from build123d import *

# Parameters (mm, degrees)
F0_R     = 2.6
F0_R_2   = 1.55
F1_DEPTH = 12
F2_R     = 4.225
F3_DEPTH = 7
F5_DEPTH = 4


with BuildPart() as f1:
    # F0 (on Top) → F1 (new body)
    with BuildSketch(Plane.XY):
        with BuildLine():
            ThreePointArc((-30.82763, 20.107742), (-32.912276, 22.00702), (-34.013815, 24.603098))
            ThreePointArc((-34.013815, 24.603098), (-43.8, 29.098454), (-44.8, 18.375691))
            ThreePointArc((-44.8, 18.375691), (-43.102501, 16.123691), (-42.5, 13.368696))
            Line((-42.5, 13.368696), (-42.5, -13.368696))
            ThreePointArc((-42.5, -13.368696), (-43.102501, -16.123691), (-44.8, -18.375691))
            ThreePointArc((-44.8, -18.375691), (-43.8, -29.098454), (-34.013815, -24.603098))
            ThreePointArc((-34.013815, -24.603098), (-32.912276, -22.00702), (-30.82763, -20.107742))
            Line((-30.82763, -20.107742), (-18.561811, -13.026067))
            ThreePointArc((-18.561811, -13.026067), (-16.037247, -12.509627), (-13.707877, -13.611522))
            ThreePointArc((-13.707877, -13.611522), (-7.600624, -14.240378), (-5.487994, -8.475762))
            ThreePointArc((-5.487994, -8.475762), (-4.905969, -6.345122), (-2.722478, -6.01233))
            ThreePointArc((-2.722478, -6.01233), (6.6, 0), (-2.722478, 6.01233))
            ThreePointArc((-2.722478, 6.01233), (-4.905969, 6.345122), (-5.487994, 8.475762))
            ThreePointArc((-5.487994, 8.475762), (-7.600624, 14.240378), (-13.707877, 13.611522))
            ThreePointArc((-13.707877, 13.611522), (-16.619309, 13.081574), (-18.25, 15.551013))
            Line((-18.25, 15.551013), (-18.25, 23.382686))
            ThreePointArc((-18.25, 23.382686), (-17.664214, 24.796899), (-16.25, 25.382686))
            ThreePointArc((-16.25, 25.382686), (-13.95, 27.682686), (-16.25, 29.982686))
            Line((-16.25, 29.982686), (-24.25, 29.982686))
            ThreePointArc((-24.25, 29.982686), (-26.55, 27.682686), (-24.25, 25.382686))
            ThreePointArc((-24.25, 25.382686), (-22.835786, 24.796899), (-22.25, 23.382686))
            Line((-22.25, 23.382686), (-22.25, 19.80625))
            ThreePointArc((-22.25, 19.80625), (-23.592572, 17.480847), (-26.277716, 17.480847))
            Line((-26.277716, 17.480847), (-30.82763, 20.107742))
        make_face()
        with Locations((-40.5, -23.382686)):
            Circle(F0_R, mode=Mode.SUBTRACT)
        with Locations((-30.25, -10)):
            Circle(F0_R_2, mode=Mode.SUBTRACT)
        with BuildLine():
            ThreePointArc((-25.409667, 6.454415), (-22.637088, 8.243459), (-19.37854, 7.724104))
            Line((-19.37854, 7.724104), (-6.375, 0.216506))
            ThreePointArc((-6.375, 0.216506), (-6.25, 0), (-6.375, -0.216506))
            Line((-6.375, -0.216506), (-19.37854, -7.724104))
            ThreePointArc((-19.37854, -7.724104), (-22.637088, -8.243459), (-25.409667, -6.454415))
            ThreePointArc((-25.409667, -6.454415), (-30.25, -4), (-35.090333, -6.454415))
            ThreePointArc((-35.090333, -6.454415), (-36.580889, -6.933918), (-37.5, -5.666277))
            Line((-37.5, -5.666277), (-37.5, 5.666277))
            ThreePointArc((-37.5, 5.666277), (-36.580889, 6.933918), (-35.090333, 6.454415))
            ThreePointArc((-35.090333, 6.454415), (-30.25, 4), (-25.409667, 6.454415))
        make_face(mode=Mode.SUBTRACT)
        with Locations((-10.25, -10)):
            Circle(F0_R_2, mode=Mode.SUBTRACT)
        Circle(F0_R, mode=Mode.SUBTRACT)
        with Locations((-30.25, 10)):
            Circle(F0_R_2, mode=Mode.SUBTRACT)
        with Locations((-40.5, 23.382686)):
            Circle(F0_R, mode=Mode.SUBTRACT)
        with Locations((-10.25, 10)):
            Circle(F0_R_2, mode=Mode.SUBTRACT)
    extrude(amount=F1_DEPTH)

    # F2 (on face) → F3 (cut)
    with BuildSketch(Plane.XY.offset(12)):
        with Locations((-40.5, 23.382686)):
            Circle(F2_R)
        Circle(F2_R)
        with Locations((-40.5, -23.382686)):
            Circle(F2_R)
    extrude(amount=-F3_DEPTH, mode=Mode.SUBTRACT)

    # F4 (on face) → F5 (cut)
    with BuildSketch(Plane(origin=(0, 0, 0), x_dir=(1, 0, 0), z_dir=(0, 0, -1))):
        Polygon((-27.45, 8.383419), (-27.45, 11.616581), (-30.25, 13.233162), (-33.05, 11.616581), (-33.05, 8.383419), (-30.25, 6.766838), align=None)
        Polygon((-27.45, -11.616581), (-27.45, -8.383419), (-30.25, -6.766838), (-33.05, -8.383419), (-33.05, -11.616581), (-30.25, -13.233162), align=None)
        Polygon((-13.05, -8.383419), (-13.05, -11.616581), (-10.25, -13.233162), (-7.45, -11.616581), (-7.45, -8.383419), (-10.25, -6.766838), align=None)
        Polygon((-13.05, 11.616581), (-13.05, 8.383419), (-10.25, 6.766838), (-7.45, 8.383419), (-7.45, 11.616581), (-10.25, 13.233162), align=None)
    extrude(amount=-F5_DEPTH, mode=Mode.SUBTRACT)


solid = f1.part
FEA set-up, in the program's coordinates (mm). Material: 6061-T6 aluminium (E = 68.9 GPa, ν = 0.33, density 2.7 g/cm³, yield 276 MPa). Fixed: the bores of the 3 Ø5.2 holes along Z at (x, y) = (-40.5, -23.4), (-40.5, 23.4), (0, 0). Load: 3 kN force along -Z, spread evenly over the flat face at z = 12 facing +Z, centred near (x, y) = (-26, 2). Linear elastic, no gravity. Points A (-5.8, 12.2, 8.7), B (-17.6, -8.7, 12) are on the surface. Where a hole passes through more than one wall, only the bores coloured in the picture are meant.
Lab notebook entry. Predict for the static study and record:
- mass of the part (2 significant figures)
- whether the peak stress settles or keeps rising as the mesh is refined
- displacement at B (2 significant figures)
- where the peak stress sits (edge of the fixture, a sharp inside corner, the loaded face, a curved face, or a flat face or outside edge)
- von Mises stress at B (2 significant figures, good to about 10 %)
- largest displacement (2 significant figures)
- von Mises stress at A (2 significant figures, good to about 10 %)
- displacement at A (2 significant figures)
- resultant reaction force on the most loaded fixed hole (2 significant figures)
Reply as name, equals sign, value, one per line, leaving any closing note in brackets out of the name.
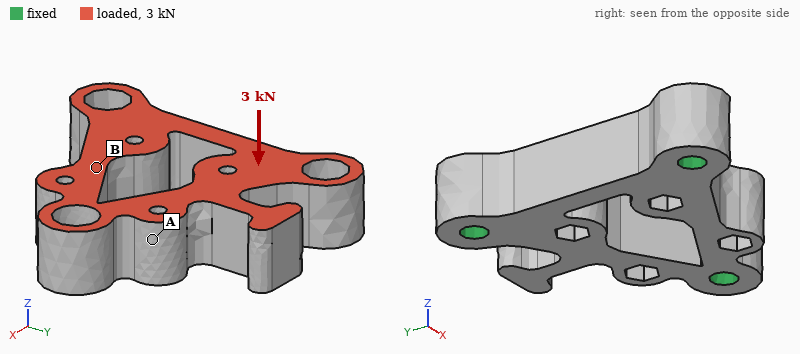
mass of the part = 40 g
whether the peak stress settles or keeps rising as the mesh is refined = keeps rising
displacement at B = 9.4 µm
where the peak stress sits = edge of the fixture
von Mises stress at B = 21 MPa
largest displacement = 29 µm
von Mises stress at A = 8.0 MPa
displacement at A = 11 µm
resultant reaction force on the most loaded fixed hole = 1.2 kN
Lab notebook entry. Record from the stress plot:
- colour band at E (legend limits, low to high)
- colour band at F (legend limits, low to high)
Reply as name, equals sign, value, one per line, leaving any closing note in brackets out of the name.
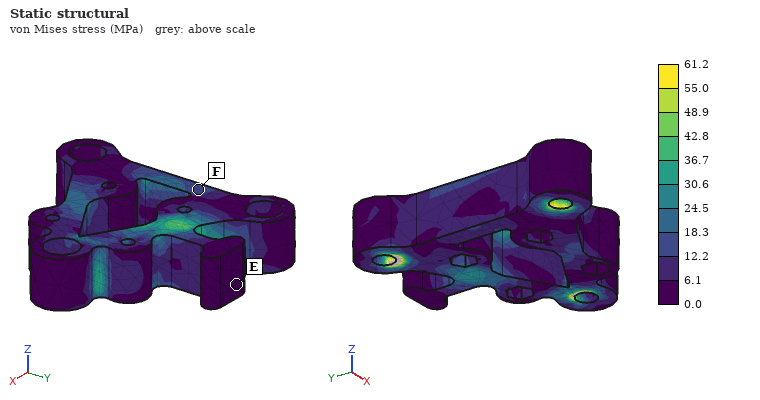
colour band at E = 0.0 to 6.1 MPa
colour band at F = 12.2 to 18.3 MPa
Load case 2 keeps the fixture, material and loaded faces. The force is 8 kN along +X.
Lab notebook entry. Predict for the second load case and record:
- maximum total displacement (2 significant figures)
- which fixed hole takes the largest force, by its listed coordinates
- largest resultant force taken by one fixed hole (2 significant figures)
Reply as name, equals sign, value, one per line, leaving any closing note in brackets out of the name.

maximum total displacement = 0.12 mm
which fixed hole takes the largest force, by its listed coordinates = (0, 0)
largest resultant force taken by one fixed hole = 3.8 kN
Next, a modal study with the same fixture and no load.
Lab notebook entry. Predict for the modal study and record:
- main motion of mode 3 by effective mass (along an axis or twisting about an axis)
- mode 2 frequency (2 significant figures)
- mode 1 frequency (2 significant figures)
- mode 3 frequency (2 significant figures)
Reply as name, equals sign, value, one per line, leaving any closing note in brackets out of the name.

main motion of mode 3 by effective mass = along X
mode 2 frequency = 9700 Hz
mode 1 frequency = 9200 Hz
mode 3 frequency = 12 kHz
